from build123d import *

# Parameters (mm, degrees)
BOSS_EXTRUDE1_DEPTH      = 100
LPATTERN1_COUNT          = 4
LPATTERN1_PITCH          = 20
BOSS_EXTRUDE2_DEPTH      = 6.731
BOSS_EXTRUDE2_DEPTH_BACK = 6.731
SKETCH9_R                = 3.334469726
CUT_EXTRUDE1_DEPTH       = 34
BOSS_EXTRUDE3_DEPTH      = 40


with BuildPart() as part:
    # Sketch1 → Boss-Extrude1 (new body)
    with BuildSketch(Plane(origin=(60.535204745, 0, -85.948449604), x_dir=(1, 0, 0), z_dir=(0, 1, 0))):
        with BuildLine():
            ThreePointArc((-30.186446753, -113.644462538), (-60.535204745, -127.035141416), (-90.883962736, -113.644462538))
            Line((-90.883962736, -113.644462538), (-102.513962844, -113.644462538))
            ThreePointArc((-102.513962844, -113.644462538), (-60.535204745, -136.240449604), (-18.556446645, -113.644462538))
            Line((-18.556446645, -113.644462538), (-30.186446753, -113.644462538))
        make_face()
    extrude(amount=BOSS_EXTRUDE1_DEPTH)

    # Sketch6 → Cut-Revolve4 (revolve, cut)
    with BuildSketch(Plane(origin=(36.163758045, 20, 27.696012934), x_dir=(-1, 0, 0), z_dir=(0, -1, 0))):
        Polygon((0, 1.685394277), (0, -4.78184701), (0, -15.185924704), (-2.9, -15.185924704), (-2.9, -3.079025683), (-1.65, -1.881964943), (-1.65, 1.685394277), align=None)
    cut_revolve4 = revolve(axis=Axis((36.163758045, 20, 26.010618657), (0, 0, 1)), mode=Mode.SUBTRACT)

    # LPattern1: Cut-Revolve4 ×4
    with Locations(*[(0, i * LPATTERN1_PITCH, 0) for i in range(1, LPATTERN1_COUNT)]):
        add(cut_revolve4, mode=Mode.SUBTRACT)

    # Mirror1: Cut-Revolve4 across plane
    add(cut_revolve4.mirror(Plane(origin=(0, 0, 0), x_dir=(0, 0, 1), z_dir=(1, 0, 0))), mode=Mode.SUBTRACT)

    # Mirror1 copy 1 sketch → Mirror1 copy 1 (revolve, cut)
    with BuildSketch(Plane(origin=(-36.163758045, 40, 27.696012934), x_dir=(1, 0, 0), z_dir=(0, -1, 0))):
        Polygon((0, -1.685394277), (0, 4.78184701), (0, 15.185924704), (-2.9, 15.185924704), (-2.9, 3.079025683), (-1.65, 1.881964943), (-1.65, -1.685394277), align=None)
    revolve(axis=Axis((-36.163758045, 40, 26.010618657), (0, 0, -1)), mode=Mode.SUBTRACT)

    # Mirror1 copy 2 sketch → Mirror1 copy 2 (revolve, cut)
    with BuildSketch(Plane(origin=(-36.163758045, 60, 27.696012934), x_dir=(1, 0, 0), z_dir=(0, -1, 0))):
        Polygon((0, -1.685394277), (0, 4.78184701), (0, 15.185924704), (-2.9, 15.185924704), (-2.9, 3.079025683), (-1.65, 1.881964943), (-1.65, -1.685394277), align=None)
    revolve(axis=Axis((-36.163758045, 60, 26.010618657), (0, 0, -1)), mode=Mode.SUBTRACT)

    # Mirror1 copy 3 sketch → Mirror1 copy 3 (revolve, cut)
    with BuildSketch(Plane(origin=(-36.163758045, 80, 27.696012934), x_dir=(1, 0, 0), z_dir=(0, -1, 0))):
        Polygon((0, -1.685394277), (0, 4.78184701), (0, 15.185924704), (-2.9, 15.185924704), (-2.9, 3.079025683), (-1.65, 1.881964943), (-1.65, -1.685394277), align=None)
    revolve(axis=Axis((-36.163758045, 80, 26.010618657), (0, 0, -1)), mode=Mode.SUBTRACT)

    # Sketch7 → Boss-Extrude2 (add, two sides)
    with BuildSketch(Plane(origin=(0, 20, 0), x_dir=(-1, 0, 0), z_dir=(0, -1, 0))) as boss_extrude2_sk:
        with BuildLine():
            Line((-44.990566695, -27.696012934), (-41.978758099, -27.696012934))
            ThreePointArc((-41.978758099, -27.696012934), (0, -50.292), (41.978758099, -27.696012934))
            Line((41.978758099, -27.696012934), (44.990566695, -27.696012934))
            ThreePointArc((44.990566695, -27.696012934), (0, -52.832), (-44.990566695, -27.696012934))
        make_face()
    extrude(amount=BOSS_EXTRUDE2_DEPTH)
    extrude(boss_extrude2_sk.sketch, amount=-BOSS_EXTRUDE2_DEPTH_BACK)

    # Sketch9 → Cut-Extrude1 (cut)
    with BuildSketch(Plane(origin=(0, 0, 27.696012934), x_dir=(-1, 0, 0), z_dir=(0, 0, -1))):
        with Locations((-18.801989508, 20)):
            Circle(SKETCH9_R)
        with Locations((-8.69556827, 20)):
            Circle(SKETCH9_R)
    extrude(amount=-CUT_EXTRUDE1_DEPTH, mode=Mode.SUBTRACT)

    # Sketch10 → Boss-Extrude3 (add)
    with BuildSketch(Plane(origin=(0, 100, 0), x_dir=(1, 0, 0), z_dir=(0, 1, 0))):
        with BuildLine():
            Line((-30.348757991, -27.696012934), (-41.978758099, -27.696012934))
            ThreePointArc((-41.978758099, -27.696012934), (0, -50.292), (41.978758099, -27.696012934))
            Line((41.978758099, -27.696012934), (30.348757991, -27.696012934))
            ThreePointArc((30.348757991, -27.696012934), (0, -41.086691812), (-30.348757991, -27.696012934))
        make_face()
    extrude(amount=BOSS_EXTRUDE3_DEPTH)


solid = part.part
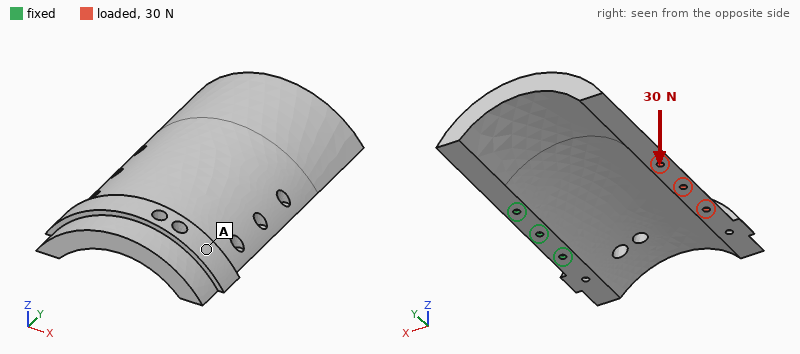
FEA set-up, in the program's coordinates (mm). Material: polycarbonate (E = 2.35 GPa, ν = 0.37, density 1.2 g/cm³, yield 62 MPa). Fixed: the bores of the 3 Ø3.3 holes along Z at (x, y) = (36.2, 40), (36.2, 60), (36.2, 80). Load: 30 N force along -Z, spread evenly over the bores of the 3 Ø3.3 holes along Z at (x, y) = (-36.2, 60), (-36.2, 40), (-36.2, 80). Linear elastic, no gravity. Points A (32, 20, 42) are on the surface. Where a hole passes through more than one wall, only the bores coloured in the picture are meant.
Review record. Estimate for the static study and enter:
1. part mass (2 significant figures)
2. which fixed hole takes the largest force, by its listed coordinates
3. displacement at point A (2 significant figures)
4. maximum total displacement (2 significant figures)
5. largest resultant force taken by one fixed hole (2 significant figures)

130 g
(36.2, 60)
0.30 mm
2.0 mm
20 N
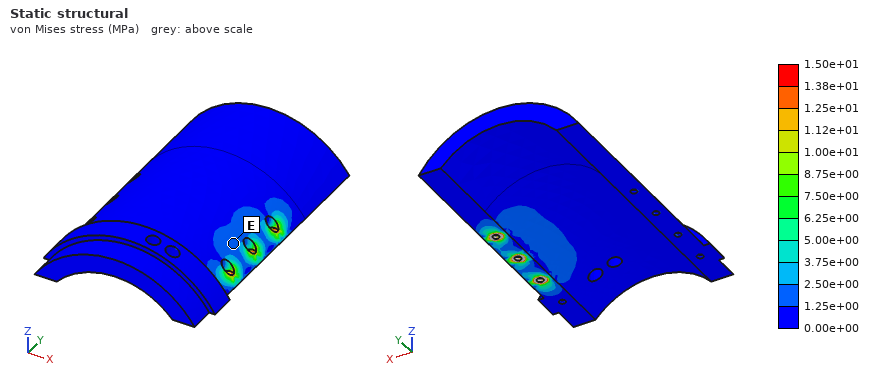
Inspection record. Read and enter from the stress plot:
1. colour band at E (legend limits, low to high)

1.25e+00 to 2.50e+00 MPa
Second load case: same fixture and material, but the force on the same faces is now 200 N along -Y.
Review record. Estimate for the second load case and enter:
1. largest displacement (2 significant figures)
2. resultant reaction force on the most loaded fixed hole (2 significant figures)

1.9 mm
350 N
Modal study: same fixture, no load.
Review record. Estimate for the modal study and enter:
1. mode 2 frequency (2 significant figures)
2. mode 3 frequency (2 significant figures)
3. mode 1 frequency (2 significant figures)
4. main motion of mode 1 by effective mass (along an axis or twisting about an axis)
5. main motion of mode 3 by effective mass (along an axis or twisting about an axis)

220 Hz
520 Hz
95 Hz
along Z
along Y
